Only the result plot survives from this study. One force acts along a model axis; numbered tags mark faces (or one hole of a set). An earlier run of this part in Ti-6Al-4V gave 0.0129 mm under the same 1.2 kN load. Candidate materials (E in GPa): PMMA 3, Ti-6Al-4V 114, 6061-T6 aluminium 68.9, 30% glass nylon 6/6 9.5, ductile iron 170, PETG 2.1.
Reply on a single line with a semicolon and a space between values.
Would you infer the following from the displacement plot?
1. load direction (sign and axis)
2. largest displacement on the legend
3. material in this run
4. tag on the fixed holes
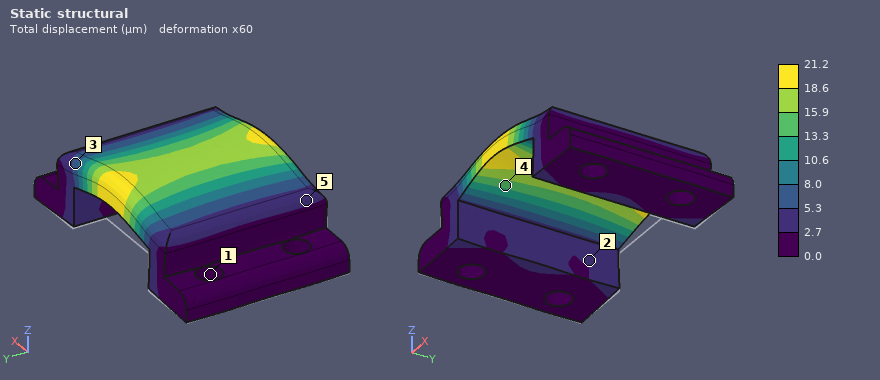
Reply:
+Z; 21.2 µm; 6061-T6 aluminium; 1
